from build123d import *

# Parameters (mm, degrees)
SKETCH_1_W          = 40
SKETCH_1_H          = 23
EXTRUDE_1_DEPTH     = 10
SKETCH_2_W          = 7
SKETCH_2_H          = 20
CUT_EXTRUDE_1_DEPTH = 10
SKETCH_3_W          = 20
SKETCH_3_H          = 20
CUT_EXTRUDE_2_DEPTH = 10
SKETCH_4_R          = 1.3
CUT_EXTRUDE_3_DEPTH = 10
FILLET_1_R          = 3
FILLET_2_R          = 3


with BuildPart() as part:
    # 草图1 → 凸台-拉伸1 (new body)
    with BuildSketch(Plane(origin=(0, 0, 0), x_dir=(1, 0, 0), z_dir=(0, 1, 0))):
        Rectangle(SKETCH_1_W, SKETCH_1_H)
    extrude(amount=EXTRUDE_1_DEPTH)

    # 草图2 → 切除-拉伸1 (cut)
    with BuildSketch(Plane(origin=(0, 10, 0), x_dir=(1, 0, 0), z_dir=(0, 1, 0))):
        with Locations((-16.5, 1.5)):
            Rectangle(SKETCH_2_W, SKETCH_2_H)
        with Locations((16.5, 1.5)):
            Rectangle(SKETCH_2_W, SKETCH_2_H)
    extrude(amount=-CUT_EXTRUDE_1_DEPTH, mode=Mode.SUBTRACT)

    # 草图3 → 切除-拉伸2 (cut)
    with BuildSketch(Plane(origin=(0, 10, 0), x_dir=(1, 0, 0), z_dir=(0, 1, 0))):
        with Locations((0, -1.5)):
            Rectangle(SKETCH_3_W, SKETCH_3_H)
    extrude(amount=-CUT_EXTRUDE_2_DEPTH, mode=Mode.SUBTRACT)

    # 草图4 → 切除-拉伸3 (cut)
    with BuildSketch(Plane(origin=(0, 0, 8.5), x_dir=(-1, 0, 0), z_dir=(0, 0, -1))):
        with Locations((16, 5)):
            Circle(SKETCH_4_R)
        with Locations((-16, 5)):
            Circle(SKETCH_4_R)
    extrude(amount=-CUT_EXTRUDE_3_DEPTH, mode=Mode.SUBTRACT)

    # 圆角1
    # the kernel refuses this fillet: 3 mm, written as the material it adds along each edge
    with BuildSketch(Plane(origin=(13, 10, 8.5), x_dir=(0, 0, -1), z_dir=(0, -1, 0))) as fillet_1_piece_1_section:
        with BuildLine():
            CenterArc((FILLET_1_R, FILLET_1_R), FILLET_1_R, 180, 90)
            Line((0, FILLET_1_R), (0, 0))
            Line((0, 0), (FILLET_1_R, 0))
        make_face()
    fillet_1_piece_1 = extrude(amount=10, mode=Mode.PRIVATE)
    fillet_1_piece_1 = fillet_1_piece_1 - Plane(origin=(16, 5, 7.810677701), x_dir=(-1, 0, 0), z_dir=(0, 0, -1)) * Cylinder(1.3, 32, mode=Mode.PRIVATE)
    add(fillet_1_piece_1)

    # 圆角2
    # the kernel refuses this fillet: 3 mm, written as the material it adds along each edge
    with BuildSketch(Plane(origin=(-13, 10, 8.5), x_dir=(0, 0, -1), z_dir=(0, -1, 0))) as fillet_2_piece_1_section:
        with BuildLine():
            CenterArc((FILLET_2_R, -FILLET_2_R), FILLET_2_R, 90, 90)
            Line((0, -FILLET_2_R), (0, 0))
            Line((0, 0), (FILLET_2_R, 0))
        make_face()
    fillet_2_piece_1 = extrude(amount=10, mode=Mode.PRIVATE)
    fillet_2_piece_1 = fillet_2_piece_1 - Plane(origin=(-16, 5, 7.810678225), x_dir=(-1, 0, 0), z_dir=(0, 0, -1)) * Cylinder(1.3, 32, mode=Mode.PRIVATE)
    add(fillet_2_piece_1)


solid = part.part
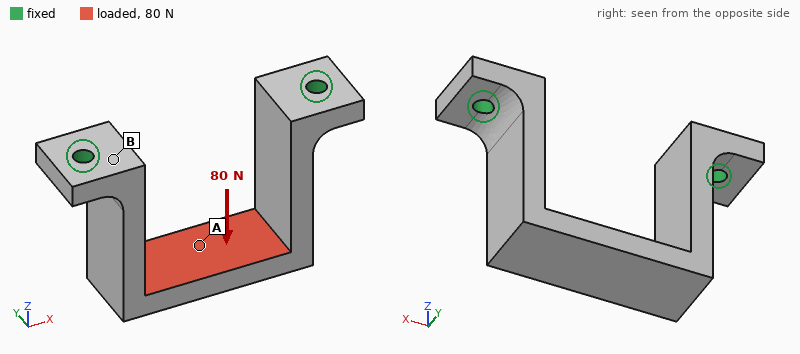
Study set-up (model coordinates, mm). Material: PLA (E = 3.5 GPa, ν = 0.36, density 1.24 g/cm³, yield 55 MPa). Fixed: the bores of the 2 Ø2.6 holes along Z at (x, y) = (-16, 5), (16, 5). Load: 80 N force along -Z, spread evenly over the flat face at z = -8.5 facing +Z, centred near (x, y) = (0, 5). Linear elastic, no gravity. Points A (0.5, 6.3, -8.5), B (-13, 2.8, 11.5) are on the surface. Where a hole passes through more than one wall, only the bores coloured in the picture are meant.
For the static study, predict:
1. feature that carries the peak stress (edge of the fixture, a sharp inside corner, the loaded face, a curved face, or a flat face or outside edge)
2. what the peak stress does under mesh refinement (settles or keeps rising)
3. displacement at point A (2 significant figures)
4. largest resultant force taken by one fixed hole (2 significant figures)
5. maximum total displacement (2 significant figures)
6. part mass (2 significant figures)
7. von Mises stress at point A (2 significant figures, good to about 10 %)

edge of the fixture
keeps rising
80 µm
42 N
86 µm
3.0 g
7.2 MPa
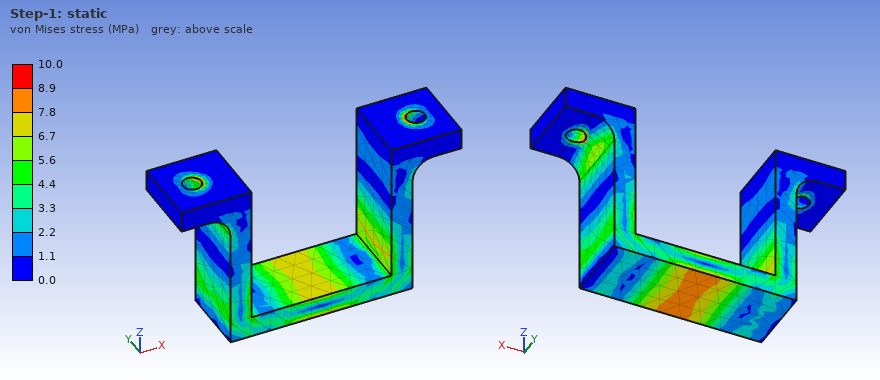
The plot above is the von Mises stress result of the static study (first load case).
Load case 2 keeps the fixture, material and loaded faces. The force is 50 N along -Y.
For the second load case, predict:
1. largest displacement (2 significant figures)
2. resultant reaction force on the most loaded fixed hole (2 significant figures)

0.30 mm
25 N
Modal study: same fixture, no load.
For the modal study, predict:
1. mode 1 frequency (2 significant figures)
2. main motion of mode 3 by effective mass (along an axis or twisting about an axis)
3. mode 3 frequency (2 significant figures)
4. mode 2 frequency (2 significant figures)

1800 Hz
twisting about Z
2900 Hz
1800 Hz
